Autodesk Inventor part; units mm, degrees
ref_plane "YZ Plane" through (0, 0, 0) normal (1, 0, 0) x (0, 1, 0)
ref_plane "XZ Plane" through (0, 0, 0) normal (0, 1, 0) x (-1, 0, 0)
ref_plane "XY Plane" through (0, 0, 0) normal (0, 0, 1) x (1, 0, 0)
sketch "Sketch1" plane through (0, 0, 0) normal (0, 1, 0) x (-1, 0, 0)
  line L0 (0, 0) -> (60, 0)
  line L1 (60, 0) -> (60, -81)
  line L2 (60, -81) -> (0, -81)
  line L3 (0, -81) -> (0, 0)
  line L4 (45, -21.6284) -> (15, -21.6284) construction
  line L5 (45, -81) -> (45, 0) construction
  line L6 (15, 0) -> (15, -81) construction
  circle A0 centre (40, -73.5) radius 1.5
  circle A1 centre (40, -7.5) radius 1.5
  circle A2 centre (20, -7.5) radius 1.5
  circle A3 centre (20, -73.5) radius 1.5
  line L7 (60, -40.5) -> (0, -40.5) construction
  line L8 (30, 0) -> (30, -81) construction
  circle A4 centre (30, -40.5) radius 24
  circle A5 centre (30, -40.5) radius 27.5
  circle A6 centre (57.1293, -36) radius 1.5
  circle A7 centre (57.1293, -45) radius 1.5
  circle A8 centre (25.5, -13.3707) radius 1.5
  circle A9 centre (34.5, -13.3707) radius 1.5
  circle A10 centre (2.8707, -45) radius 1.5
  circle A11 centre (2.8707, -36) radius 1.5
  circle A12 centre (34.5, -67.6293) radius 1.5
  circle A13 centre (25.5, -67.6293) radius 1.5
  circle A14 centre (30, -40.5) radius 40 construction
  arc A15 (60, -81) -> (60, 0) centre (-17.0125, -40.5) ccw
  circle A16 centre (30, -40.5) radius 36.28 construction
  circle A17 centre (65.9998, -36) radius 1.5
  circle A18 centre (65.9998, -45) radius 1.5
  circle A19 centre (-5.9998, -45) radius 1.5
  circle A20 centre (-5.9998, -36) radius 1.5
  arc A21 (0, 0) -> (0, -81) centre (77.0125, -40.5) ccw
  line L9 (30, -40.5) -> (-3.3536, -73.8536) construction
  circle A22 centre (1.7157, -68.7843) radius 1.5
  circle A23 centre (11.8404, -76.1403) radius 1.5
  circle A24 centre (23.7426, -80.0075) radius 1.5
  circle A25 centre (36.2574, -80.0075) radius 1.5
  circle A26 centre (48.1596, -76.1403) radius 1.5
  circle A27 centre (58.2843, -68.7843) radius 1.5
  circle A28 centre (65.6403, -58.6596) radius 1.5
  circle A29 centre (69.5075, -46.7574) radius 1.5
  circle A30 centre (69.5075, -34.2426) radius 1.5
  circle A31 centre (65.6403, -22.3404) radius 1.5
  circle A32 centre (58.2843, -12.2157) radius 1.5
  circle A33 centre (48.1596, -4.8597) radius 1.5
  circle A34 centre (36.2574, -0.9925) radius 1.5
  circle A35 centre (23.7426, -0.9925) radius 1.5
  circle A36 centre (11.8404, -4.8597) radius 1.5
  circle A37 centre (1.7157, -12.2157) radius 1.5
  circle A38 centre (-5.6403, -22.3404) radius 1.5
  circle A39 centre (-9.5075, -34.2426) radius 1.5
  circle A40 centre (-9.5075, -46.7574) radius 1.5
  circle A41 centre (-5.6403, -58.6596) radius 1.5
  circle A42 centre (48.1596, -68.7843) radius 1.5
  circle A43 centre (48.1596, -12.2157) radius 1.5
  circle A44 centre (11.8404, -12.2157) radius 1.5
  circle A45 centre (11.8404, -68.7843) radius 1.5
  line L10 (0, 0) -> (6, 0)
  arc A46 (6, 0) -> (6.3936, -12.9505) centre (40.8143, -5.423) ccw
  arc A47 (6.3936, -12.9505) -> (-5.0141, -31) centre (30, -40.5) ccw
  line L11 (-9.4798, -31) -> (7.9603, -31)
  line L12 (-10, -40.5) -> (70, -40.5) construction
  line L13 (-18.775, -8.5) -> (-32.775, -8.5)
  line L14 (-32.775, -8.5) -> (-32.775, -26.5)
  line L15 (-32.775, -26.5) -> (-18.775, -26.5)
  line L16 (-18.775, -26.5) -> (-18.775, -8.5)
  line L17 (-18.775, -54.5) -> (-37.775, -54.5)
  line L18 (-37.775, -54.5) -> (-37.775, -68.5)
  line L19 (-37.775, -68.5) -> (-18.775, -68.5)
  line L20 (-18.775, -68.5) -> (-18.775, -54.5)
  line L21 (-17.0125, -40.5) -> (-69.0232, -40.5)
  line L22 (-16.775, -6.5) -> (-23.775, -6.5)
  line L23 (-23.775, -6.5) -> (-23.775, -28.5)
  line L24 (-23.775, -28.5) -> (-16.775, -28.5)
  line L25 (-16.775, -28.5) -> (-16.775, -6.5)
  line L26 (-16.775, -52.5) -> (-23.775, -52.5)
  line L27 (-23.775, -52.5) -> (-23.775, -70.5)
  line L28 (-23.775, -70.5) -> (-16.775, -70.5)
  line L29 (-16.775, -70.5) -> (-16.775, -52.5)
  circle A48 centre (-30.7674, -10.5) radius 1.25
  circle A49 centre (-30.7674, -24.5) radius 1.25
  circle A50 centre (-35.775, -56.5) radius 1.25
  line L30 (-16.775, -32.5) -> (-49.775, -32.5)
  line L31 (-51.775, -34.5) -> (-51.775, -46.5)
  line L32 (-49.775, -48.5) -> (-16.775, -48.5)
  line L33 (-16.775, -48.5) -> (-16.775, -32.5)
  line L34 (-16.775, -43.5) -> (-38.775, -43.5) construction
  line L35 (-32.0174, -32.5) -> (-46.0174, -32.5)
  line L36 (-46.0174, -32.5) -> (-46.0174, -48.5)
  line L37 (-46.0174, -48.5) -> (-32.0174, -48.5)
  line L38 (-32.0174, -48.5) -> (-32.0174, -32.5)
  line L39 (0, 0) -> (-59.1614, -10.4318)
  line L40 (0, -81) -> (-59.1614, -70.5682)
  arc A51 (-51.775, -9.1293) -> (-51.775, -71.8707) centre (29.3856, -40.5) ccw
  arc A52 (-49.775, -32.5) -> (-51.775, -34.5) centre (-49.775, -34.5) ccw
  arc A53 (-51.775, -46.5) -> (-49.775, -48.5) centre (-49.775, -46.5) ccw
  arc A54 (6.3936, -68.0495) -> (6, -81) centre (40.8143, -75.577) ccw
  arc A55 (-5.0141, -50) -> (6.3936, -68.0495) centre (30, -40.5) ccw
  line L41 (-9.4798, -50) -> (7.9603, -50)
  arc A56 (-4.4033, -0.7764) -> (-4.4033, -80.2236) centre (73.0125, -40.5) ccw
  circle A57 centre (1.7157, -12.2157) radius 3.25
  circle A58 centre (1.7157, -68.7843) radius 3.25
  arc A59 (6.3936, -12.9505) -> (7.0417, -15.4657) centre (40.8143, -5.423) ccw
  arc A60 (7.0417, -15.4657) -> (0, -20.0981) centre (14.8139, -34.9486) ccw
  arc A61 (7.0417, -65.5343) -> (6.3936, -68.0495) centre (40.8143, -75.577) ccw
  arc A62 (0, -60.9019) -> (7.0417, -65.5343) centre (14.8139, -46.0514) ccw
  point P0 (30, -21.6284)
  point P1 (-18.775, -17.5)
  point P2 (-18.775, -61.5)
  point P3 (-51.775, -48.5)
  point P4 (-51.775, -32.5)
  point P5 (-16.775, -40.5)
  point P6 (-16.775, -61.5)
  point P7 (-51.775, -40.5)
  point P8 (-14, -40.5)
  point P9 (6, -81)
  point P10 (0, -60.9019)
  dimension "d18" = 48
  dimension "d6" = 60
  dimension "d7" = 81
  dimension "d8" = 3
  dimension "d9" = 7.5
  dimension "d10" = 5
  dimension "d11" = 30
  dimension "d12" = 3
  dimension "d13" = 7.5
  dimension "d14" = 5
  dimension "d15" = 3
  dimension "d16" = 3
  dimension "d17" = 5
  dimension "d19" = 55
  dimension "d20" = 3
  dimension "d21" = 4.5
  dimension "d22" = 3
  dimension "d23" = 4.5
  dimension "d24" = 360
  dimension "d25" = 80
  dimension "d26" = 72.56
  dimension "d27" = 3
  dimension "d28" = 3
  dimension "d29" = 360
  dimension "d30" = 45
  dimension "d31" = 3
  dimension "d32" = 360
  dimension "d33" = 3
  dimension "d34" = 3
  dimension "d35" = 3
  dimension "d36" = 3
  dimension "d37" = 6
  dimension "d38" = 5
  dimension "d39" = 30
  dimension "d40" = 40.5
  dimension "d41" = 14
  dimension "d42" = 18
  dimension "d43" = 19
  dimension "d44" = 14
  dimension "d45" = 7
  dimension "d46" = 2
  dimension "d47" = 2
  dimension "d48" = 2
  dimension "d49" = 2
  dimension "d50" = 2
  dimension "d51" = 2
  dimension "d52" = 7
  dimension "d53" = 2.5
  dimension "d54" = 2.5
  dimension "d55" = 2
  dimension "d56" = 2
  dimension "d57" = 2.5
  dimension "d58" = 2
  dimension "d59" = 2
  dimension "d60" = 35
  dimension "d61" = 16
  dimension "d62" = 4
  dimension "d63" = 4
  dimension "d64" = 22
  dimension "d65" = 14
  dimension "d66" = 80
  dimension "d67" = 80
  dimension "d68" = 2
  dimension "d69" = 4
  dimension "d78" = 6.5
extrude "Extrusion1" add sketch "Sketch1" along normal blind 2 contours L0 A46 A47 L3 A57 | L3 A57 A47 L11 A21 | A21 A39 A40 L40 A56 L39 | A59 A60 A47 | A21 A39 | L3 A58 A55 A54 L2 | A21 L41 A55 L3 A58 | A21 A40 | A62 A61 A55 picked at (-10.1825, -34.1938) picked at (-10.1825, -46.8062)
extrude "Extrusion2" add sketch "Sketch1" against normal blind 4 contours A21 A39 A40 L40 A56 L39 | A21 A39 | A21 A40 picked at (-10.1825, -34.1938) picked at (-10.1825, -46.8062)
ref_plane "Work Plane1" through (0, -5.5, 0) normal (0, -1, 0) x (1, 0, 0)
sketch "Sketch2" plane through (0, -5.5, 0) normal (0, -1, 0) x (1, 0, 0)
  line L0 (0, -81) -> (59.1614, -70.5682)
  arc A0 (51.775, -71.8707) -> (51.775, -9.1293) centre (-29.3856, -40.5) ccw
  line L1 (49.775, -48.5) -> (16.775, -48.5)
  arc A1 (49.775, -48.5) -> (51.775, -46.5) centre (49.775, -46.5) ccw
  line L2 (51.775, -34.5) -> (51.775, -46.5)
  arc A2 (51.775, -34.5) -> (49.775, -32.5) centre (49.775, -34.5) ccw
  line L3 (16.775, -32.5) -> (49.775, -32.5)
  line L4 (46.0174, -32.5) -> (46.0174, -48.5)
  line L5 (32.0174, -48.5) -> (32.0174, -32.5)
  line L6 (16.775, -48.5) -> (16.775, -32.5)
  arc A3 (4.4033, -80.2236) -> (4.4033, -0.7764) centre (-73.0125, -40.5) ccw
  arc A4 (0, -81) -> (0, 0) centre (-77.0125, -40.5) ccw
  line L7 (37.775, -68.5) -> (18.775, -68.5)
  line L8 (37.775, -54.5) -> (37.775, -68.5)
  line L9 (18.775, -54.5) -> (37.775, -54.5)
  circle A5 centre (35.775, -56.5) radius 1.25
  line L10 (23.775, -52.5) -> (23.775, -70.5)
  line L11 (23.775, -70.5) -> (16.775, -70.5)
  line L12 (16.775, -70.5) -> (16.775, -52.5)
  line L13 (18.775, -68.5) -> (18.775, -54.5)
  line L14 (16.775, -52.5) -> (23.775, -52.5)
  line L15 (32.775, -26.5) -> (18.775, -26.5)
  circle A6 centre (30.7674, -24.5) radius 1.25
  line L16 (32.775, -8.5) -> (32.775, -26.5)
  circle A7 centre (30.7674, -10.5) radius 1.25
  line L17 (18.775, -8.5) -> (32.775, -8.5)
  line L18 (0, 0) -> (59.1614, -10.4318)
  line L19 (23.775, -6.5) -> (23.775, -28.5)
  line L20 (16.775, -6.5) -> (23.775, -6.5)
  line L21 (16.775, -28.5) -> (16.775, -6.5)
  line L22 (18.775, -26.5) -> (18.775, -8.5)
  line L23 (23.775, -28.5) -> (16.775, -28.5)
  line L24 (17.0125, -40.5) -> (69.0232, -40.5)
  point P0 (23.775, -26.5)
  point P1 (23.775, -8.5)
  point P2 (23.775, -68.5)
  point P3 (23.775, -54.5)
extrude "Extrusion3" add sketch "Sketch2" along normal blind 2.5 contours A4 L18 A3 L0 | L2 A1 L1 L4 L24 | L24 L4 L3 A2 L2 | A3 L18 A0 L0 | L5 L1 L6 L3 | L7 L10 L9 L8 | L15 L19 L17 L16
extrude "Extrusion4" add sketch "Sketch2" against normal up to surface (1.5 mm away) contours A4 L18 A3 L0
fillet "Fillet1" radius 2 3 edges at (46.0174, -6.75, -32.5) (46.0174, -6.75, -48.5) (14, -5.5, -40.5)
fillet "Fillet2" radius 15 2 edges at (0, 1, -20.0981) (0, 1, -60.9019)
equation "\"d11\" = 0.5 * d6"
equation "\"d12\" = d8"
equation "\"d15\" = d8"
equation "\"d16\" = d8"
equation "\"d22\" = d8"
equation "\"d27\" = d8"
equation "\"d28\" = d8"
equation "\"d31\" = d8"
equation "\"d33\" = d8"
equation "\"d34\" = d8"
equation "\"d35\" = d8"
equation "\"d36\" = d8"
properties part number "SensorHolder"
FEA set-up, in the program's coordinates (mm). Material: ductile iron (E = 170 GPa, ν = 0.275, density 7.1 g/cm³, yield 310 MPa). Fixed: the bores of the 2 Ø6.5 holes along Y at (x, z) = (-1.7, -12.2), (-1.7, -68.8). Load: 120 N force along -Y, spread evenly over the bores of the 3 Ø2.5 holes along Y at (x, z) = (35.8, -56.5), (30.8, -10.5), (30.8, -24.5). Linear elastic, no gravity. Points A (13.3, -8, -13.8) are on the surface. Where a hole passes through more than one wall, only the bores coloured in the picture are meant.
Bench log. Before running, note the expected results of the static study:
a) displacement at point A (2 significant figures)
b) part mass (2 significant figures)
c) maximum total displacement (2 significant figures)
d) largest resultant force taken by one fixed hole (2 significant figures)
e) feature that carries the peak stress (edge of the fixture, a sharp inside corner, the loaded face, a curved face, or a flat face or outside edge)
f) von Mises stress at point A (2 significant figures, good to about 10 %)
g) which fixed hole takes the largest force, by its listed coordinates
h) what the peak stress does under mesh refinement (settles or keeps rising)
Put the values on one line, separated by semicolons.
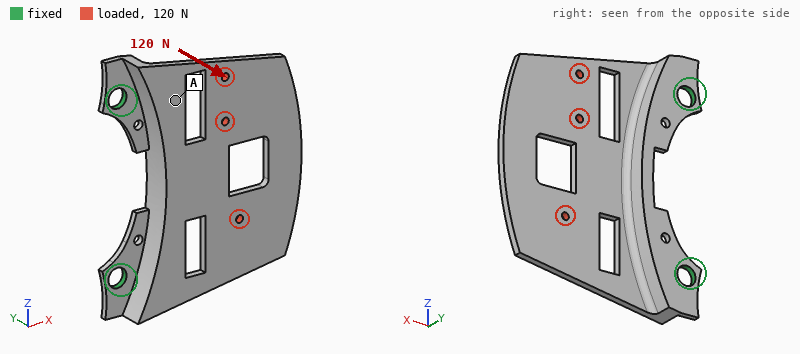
0.052 mm; 75 g; 0.33 mm; 110 N; edge of the fixture; 21 MPa; (-1.7, -12.2); keeps rising
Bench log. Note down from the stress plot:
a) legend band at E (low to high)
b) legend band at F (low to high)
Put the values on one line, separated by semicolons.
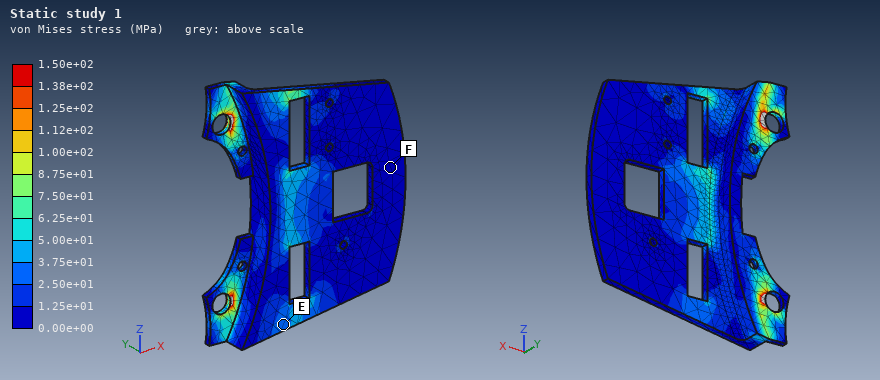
2.50e+01 to 3.75e+01 MPa; 0.00e+00 to 1.25e+01 MPa
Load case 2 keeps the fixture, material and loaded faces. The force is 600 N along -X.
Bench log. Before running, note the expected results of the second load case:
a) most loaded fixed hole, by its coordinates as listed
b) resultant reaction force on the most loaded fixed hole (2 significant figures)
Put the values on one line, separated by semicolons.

(-1.7, -12.2); 410 N
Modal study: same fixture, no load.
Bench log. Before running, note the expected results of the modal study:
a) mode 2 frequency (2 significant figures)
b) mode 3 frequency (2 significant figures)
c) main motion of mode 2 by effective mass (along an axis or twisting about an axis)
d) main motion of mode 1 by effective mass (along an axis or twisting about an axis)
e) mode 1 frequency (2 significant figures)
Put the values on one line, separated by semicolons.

1400 Hz; 2500 Hz; twisting about X; along Y; 530 Hz
